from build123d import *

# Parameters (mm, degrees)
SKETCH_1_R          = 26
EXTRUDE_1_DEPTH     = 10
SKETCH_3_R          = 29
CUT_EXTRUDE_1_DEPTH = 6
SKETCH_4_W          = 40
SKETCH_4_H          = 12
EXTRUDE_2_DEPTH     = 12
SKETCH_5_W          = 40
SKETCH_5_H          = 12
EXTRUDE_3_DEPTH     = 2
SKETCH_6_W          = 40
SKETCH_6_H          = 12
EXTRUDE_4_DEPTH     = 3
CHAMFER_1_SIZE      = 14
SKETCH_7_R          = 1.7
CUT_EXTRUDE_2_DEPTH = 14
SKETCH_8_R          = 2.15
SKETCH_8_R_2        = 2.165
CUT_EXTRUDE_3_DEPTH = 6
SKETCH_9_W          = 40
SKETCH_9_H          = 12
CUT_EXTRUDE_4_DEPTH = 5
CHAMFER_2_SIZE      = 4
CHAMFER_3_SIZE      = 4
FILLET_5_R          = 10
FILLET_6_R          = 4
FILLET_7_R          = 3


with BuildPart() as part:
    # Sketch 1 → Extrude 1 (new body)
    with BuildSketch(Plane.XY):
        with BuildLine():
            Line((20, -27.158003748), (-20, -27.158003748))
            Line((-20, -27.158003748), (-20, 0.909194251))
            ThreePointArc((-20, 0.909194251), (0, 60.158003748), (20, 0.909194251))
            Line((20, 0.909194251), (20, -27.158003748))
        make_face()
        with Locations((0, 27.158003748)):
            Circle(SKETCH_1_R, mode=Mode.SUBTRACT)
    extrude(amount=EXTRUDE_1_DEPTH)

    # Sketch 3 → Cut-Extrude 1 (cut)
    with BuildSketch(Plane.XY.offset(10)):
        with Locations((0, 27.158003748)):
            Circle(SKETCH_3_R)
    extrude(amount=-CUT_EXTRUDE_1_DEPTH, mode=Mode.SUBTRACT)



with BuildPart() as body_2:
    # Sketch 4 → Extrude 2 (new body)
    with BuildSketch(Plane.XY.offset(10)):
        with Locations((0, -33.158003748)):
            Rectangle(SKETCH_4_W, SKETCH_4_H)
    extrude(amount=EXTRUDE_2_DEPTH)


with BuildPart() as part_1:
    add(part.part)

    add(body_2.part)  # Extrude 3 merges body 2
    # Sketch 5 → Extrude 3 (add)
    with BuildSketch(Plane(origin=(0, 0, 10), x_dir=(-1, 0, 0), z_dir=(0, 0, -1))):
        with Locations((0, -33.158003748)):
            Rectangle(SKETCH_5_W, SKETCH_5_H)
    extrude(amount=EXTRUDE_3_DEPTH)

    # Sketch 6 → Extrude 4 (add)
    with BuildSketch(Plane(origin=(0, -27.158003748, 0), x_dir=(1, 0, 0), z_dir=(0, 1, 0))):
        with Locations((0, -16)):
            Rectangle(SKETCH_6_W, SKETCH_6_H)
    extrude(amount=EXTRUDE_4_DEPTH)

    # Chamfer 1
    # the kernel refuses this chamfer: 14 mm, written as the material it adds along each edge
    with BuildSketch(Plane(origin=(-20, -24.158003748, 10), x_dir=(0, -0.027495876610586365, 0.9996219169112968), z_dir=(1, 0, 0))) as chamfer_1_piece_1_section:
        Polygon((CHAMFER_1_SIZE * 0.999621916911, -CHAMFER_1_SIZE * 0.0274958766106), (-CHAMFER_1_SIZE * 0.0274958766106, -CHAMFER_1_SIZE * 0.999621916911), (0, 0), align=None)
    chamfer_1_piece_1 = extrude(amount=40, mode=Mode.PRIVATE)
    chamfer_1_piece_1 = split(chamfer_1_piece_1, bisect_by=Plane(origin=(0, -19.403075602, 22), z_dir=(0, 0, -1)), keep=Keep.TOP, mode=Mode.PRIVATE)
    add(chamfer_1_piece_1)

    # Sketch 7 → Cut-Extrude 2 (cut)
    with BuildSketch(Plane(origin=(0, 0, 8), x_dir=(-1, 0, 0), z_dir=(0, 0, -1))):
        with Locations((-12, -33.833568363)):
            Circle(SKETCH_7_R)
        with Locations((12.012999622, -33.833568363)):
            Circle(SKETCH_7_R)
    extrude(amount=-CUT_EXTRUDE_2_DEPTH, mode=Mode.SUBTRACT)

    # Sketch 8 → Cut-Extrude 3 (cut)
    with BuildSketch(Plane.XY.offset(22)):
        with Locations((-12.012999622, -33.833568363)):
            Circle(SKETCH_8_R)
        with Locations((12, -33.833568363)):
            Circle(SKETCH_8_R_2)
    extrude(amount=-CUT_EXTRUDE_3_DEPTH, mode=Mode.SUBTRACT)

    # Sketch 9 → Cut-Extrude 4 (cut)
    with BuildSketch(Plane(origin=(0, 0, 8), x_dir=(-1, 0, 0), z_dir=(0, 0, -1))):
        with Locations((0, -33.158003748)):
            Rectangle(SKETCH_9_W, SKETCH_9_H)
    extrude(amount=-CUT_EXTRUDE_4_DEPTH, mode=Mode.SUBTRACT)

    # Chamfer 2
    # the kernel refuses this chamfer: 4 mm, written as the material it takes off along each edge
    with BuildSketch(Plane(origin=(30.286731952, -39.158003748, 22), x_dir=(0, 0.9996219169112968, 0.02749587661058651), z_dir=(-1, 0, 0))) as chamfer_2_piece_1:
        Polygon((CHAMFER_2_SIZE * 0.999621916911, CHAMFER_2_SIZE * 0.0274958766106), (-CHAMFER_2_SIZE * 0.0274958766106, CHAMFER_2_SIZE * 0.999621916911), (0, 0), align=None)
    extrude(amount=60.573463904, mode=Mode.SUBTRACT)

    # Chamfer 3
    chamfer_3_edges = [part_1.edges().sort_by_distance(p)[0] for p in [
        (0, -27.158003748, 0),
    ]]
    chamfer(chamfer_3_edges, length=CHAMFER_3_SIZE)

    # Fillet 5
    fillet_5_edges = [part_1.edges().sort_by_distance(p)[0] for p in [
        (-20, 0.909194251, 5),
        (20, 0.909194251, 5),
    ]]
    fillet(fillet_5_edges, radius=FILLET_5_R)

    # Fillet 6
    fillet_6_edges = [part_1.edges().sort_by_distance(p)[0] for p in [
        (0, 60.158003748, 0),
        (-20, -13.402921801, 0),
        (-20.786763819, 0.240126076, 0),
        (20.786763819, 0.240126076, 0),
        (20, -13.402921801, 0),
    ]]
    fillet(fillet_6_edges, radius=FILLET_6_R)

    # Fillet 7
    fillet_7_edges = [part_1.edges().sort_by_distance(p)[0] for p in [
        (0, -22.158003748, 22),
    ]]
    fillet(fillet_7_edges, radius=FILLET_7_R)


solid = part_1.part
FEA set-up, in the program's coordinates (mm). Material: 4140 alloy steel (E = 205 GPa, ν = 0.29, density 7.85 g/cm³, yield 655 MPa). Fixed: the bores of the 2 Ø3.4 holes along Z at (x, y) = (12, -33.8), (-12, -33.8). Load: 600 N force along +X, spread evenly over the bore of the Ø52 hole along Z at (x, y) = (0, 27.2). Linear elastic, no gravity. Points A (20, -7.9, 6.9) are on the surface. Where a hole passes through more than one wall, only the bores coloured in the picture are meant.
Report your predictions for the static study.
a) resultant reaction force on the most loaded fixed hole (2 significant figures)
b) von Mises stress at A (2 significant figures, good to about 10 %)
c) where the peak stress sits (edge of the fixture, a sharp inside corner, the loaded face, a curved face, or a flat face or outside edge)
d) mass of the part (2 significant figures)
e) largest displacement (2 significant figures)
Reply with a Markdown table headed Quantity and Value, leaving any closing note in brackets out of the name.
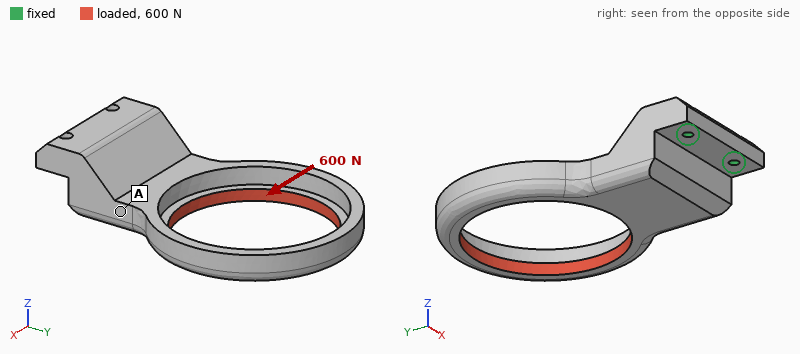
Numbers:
| Quantity | Value |
|---|---|
| resultant reaction force on the most loaded fixed hole | 1.5 kN |
| von Mises stress at A | 19 MPa |
| where the peak stress sits | edge of the fixture |
| mass of the part | 210 g |
| largest displacement | 0.13 mm |
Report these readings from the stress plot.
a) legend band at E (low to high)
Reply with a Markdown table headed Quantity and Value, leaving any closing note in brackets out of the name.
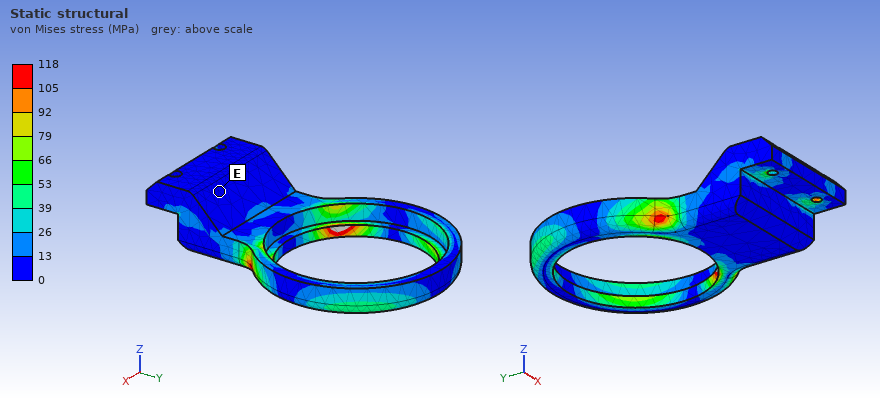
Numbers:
| Quantity | Value |
|---|---|
| legend band at E | 0 to 13 MPa |
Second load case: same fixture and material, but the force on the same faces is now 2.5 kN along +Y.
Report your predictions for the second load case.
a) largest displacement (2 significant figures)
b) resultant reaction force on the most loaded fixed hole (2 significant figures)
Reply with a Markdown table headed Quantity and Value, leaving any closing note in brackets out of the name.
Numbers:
| Quantity | Value |
|---|---|
| largest displacement | 0.38 mm |
| resultant reaction force on the most loaded fixed hole | 1.3 kN |
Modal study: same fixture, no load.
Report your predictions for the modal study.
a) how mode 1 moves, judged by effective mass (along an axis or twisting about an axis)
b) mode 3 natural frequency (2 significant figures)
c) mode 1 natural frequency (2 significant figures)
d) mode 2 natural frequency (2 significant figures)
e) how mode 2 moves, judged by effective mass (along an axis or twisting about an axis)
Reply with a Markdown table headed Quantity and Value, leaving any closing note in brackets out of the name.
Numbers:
| Quantity | Value |
|---|---|
| how mode 1 moves, judged by effective mass | along Z |
| mode 3 natural frequency | 2400 Hz |
| mode 1 natural frequency | 710 Hz |
| mode 2 natural frequency | 1400 Hz |
| how mode 2 moves, judged by effective mass | along X |
